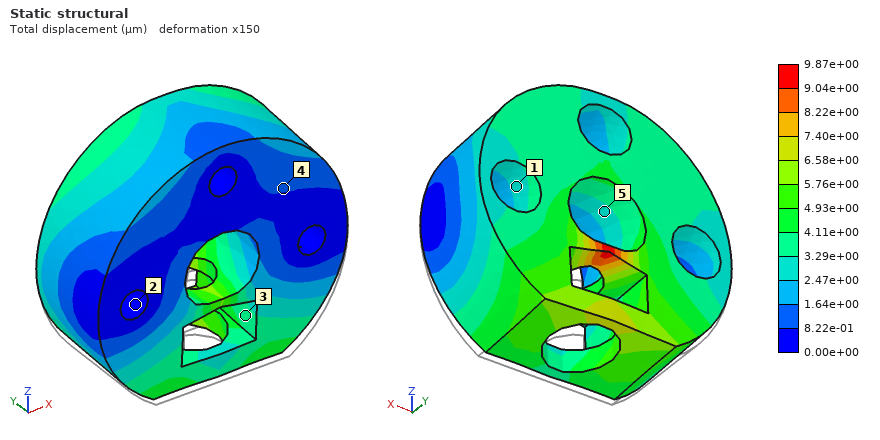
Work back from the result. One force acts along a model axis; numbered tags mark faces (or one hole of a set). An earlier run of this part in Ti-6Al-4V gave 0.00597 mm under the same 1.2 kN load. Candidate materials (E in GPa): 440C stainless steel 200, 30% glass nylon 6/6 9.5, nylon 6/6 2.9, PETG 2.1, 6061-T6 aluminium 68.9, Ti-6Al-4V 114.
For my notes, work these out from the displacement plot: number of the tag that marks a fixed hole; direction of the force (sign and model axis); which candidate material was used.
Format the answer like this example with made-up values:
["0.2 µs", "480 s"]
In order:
["2", "+Z", "6061-T6 aluminium"]
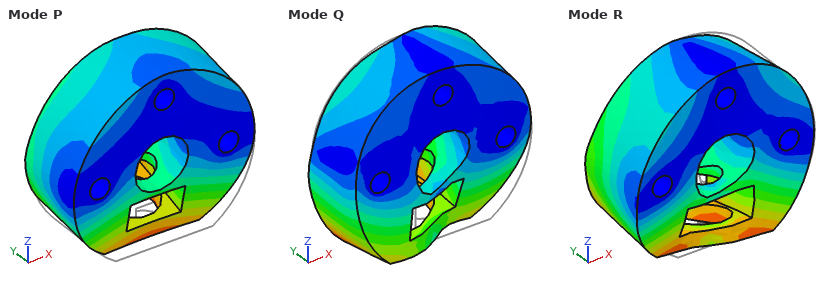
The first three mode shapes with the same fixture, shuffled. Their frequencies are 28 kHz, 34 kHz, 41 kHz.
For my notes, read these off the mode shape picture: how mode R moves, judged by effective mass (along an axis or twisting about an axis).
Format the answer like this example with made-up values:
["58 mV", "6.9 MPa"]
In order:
["along X"]
